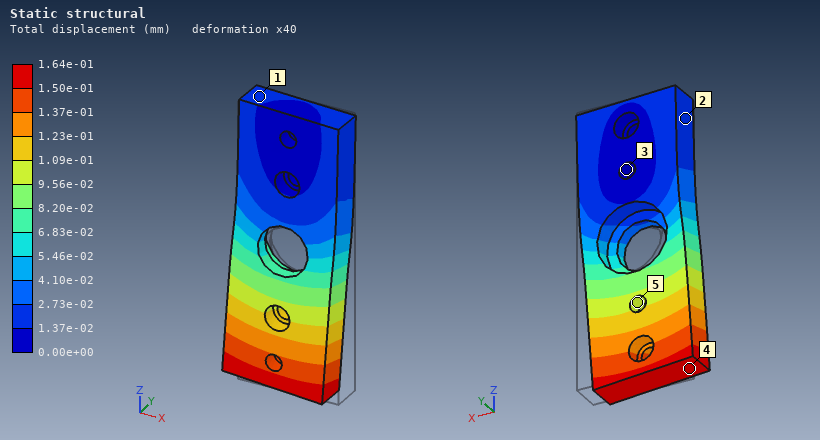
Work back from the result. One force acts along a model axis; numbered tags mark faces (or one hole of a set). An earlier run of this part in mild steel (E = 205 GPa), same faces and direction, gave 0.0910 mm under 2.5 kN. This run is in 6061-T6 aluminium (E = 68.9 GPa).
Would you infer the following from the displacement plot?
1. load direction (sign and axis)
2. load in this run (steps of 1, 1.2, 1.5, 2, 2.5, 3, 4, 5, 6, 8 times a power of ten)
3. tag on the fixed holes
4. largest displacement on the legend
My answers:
-X
1.5 kN
3
1.64e-01 mm
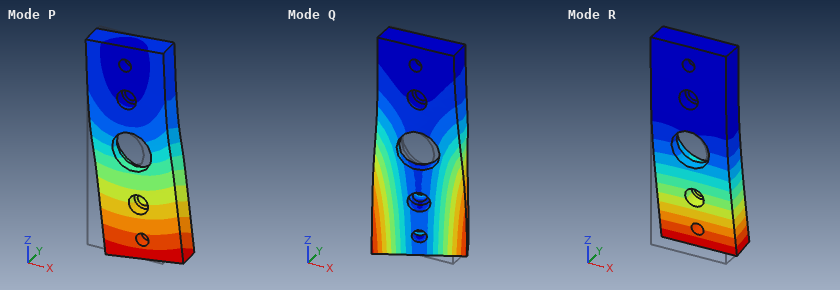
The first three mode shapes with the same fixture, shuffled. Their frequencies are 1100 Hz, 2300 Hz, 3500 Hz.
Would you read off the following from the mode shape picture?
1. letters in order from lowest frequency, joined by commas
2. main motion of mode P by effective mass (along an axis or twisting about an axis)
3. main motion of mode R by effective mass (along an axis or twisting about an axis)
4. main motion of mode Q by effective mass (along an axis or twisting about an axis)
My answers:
R, P, Q
along X
along Y
twisting about Z
